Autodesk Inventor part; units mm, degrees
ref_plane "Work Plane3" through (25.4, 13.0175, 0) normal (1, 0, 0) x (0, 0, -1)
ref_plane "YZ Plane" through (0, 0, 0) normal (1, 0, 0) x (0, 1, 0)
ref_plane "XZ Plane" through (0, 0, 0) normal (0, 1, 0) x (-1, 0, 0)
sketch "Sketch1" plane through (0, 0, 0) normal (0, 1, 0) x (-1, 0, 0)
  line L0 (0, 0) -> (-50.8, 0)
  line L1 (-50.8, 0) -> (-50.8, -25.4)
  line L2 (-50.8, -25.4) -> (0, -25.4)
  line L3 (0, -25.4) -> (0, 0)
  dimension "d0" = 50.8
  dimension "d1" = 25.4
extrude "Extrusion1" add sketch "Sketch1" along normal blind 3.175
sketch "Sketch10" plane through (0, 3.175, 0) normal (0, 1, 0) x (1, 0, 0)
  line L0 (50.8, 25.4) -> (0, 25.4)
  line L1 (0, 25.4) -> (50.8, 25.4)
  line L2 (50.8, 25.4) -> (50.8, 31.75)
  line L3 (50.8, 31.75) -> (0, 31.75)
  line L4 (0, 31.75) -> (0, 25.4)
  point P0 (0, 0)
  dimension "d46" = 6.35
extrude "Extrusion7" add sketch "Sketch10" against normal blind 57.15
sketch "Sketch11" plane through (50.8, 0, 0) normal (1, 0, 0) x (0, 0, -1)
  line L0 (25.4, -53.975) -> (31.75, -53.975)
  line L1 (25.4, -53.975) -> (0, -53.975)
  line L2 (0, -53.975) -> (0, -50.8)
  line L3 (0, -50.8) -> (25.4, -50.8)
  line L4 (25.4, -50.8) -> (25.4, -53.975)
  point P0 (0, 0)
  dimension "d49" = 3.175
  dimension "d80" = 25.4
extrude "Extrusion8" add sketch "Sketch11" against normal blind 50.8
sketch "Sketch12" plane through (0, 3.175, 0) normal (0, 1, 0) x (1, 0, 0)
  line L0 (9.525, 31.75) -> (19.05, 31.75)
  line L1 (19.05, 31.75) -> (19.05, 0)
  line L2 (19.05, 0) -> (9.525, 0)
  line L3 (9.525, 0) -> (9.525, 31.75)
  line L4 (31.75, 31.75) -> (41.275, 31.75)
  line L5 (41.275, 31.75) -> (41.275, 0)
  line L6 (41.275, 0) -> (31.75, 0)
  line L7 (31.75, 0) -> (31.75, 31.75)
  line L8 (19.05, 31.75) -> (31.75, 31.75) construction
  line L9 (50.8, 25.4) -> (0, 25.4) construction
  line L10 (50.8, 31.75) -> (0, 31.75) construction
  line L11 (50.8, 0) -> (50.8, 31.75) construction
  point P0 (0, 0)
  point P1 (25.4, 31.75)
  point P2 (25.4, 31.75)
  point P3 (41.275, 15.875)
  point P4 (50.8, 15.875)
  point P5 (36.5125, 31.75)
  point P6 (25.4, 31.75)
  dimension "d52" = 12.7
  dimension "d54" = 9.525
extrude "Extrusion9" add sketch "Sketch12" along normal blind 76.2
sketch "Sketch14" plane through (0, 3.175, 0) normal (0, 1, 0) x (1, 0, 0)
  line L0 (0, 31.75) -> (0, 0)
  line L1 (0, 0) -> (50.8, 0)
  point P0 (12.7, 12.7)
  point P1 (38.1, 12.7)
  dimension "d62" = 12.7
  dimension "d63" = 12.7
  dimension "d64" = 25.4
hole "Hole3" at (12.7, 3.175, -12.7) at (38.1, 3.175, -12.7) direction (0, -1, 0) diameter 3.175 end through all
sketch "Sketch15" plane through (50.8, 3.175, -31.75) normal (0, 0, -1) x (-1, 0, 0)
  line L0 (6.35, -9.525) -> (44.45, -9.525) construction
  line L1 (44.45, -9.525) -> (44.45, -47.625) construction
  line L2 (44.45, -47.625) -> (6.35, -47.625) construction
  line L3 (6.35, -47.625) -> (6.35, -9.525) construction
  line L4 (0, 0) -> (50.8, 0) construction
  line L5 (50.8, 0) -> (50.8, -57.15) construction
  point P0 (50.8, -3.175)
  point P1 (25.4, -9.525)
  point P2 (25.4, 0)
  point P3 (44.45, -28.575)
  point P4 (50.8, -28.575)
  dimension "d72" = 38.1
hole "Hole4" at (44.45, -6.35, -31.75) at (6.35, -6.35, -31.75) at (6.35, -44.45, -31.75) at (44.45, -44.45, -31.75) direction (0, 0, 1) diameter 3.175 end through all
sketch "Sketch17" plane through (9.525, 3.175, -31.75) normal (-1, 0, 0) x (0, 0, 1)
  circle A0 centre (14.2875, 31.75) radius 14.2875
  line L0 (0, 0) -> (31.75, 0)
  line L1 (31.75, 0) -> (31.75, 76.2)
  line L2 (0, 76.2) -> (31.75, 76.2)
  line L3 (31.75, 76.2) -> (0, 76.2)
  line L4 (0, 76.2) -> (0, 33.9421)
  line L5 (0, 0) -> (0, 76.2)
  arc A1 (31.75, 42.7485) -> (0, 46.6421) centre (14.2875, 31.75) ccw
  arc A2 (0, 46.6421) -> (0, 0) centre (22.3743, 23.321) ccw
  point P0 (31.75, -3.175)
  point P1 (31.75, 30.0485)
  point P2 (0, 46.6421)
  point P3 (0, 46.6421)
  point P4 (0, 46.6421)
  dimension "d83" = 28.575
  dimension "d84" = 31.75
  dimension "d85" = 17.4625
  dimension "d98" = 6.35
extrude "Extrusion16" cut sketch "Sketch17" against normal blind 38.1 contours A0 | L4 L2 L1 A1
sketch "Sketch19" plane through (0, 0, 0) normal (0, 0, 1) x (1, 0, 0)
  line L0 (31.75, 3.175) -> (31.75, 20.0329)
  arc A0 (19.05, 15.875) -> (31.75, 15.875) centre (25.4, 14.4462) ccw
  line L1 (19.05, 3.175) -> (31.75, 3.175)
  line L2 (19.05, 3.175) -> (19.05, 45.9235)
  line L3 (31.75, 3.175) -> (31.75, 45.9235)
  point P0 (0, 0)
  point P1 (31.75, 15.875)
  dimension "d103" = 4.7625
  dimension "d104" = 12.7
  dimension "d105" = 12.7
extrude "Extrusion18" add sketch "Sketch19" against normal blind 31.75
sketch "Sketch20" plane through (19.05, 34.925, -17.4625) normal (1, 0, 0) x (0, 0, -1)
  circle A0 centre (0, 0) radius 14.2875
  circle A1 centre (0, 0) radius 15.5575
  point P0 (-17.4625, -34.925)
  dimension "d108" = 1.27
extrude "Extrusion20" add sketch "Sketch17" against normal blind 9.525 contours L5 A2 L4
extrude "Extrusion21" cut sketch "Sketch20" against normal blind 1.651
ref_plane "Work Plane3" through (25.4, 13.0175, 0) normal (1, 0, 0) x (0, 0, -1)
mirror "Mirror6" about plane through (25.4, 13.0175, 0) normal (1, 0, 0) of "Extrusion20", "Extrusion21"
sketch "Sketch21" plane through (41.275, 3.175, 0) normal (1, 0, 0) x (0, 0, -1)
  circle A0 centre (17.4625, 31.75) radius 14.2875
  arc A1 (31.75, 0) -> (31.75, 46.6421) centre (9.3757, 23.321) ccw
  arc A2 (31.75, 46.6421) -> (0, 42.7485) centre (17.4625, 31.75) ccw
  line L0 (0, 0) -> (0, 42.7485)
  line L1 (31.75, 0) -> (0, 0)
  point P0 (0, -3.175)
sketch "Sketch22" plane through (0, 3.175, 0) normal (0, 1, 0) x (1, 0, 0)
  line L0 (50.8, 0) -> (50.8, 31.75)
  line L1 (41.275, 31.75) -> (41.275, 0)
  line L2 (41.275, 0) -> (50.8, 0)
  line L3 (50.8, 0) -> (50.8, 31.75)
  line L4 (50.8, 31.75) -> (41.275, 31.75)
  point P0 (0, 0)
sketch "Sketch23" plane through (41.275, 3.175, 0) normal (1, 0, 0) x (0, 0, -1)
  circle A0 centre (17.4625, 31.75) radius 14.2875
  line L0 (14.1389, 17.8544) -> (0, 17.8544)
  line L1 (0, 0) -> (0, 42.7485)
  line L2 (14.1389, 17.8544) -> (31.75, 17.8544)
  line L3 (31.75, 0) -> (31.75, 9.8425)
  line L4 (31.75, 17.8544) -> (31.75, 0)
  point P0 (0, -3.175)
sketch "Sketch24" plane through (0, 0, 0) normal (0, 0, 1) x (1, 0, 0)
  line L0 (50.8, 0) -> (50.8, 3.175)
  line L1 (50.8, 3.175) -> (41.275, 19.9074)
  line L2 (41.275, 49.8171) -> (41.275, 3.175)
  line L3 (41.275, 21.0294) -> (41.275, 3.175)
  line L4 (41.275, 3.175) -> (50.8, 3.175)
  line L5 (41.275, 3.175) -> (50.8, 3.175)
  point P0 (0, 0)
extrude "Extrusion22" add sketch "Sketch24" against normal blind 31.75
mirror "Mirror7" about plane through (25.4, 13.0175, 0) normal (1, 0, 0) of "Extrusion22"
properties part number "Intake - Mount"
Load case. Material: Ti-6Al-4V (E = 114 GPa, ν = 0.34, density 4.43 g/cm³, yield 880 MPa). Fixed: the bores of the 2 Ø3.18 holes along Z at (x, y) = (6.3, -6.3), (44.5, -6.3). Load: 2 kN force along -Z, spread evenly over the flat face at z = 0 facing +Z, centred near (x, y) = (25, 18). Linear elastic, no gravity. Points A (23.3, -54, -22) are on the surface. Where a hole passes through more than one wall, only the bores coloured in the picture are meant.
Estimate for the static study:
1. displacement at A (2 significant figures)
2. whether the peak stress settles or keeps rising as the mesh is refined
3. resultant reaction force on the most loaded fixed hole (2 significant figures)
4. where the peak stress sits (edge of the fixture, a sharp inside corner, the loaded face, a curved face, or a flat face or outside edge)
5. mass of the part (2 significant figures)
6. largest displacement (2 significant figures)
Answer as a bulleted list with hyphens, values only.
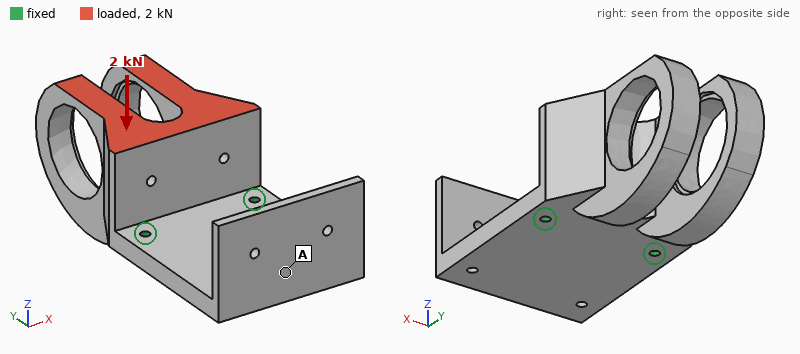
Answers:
- 0.076 mm
- keeps rising
- 1.0 kN
- edge of the fixture
- 260 g
- 0.28 mm
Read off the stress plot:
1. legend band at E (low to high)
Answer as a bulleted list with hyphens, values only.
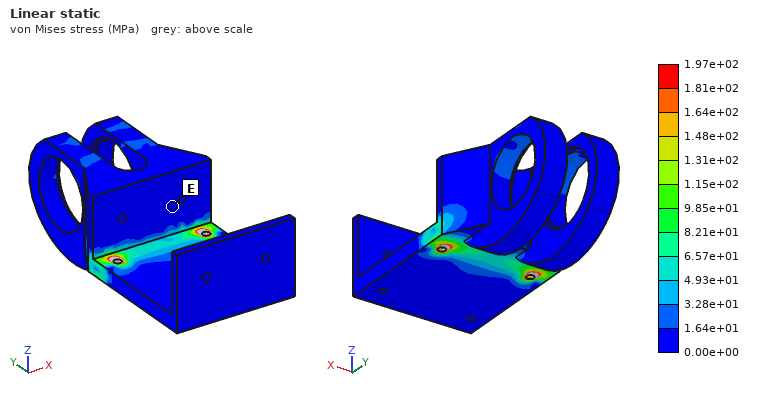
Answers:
- 0.00e+00 to 1.64e+01 MPa
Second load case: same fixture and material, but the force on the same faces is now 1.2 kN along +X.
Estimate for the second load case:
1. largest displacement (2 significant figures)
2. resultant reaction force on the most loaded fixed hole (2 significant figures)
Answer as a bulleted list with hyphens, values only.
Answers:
- 30 µm
- 1.3 kN
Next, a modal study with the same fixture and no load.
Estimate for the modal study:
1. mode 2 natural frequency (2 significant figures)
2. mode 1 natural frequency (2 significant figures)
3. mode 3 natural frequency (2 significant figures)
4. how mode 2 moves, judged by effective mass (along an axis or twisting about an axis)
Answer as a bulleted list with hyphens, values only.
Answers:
- 1600 Hz
- 1200 Hz
- 3000 Hz
- along Z
